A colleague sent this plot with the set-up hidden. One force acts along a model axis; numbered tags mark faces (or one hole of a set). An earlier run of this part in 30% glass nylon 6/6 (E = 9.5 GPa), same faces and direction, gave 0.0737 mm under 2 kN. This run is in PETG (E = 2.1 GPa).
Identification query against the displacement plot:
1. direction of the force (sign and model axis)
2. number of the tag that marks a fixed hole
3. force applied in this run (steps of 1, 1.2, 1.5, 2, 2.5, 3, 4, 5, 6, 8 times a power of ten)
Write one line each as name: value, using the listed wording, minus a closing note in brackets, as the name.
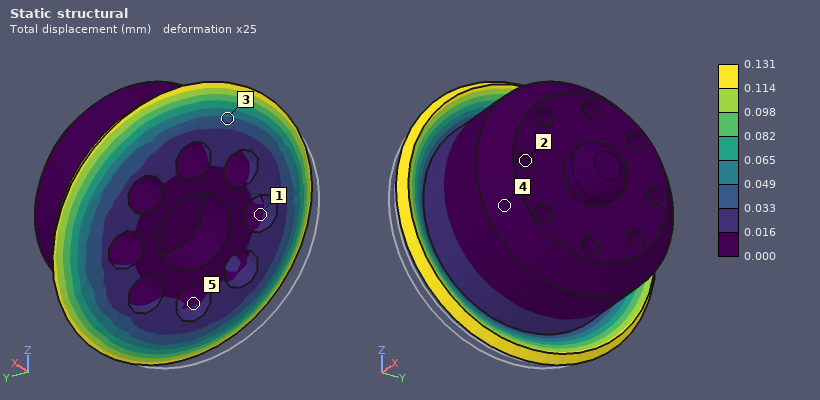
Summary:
direction of the force: +X
number of the tag that marks a fixed hole: 2
force applied in this run: 800 N
